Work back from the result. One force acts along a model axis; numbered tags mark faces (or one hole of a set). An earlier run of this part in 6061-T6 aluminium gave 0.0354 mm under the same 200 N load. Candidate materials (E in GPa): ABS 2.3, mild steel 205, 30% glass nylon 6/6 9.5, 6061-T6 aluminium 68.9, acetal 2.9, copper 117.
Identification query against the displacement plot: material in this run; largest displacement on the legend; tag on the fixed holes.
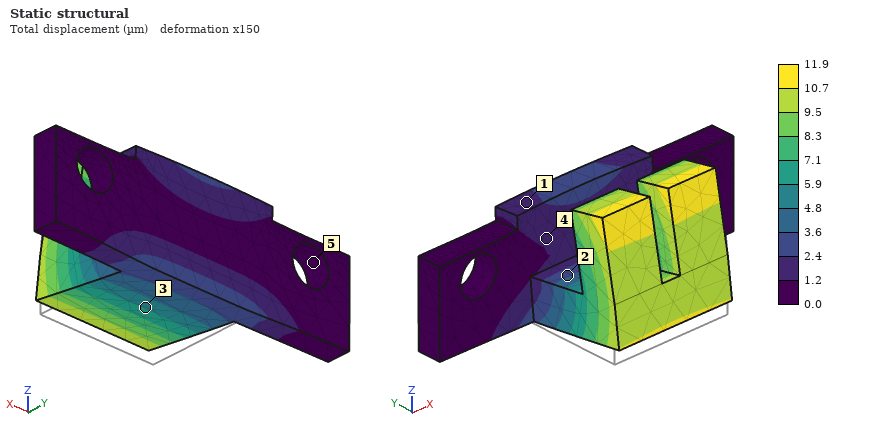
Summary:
mild steel
11.9 µm
5
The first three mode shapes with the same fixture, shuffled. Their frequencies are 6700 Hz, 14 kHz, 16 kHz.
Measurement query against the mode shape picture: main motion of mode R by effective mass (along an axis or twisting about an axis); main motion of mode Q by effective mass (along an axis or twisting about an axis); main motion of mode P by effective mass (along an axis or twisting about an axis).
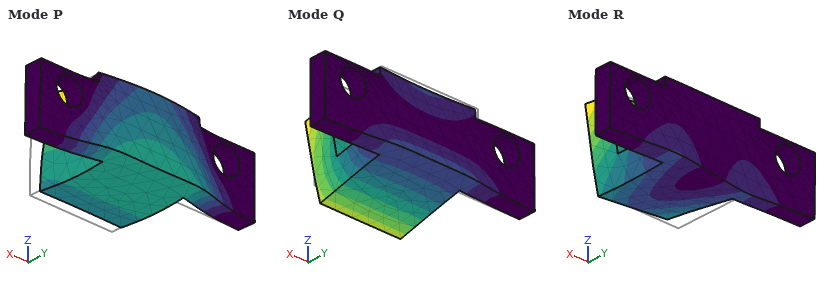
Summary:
along X
along Z
along Y
